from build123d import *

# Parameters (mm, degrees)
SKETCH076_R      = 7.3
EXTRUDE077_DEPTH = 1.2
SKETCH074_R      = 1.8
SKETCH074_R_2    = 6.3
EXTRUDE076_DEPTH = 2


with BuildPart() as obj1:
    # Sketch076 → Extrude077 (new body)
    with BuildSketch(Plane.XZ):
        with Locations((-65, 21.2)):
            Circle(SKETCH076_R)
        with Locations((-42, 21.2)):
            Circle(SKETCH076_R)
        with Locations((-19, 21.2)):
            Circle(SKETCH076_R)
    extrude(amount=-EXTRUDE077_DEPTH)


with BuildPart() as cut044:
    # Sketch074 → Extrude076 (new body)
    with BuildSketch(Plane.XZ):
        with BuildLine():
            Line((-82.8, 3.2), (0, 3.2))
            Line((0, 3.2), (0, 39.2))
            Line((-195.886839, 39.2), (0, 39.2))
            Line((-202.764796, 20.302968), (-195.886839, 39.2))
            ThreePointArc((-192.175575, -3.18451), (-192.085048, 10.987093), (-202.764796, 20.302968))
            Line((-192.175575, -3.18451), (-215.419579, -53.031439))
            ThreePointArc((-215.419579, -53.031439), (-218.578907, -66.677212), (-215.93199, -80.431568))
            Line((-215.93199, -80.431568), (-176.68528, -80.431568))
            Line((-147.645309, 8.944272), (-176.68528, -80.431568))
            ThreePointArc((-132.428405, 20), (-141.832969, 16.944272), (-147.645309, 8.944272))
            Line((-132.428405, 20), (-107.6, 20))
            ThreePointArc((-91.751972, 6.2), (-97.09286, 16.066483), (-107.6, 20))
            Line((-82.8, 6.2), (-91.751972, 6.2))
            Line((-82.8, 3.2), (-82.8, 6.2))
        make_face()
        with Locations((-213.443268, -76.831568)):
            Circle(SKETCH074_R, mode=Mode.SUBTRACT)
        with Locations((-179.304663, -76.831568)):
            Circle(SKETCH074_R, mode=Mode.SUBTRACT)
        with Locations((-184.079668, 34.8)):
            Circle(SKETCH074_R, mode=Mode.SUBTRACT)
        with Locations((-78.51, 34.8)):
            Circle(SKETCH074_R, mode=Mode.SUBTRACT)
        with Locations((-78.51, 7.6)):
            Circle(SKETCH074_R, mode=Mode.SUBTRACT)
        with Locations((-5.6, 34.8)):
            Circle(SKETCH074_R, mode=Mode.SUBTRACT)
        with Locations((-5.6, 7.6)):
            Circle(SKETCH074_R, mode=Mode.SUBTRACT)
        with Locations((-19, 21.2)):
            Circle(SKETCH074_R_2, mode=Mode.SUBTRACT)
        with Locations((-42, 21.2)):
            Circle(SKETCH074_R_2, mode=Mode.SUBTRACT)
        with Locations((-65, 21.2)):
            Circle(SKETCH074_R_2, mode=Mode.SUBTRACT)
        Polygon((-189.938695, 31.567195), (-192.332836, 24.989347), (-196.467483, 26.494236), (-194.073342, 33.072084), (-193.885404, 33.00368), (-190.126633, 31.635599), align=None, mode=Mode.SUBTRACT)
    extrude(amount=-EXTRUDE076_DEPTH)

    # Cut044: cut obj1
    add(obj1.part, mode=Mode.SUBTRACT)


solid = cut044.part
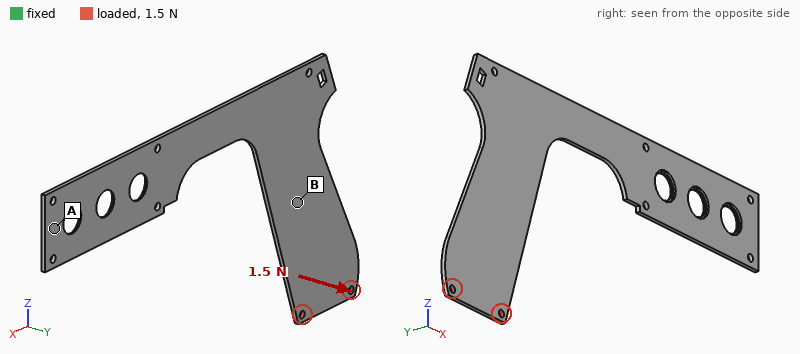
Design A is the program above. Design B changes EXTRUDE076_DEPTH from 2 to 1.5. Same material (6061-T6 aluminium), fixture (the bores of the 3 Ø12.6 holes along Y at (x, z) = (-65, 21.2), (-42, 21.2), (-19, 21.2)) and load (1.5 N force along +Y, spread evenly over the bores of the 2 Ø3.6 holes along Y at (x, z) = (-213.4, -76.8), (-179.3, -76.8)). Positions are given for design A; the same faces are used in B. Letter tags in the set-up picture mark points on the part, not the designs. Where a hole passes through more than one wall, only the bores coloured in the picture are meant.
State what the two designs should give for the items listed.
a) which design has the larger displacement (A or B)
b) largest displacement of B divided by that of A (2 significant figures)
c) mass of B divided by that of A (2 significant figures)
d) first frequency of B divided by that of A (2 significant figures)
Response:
B
2.4
0.75
0.75
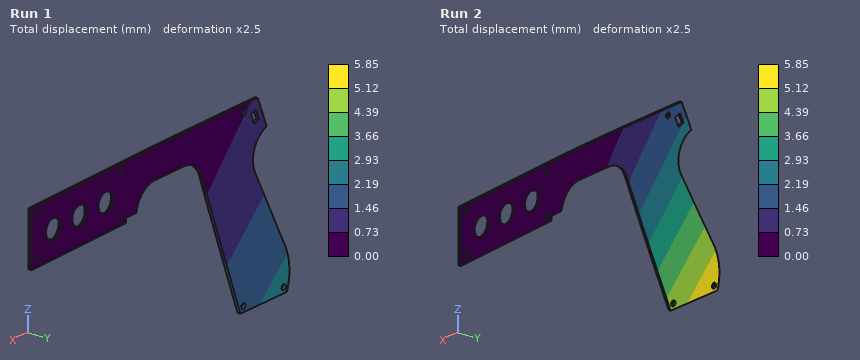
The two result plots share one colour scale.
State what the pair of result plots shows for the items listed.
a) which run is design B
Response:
Run 2
